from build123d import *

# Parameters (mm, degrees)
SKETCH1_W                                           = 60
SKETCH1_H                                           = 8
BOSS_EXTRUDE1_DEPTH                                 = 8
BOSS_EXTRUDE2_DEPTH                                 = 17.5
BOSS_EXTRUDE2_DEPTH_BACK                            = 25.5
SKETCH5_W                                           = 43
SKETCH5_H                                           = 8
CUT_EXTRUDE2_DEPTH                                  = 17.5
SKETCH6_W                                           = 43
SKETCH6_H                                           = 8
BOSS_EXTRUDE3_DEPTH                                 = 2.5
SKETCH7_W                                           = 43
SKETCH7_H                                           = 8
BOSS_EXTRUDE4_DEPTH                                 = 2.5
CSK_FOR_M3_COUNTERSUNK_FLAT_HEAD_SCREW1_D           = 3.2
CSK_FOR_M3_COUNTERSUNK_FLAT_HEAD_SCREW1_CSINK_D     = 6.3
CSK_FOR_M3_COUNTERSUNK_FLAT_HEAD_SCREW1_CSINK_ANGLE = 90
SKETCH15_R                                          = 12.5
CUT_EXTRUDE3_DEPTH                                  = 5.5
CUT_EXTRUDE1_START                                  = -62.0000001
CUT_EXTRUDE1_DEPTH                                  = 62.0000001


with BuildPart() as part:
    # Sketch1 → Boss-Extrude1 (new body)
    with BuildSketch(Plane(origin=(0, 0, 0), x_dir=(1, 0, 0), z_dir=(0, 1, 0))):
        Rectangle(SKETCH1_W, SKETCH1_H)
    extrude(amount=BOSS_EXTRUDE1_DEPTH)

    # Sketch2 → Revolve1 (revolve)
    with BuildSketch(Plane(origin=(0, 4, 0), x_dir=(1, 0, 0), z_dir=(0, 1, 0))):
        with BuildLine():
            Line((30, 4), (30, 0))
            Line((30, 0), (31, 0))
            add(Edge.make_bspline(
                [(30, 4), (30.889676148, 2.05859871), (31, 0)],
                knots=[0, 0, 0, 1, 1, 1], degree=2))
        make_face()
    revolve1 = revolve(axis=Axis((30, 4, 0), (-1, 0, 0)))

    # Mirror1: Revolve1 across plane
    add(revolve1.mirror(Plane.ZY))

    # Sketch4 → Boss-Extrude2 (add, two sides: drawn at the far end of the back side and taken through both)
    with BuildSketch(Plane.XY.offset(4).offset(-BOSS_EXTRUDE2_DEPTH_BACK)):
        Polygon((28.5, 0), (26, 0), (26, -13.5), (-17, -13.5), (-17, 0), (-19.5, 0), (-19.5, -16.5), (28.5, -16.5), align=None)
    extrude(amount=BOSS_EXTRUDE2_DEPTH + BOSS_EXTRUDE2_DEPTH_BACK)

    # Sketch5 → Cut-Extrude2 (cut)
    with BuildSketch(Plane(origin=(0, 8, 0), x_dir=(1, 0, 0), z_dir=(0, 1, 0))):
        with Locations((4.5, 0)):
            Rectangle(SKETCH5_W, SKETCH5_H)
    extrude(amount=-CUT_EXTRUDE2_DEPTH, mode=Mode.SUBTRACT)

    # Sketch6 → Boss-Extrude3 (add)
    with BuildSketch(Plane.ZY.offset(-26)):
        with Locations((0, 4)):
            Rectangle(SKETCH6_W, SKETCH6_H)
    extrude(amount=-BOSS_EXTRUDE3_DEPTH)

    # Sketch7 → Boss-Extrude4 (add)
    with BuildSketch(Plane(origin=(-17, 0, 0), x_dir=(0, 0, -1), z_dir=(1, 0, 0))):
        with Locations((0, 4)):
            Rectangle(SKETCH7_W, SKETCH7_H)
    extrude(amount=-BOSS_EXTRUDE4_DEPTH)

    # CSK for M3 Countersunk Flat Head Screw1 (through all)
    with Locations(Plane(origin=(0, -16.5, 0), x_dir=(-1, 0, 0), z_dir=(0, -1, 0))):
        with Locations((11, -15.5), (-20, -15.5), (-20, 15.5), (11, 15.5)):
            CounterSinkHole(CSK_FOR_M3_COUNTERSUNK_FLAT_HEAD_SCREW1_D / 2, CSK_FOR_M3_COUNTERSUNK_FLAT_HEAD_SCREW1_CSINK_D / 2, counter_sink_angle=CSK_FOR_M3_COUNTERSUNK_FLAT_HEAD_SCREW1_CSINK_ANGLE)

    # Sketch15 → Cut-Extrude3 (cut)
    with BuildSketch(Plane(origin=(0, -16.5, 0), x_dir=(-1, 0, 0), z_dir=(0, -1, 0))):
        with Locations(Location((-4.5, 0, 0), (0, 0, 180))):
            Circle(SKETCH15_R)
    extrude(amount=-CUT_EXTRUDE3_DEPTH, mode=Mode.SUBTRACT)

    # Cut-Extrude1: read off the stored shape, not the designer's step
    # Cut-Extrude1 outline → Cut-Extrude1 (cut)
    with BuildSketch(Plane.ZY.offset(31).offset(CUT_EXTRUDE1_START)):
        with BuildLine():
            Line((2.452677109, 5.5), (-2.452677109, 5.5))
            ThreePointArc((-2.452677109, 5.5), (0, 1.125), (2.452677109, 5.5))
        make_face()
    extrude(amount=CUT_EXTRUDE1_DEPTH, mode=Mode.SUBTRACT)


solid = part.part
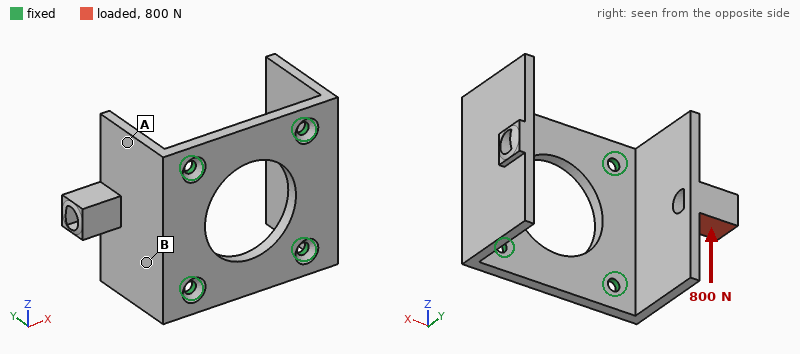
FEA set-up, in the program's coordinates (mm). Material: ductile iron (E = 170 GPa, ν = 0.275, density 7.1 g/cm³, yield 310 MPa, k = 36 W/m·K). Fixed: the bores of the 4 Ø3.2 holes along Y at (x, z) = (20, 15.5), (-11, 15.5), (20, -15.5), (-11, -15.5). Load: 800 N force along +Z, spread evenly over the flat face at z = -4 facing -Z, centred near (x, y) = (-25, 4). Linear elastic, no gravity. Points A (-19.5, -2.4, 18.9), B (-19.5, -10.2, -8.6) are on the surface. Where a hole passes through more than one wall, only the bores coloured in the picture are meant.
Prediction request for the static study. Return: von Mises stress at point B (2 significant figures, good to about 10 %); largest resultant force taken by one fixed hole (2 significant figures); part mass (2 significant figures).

56 MPa
670 N
68 g
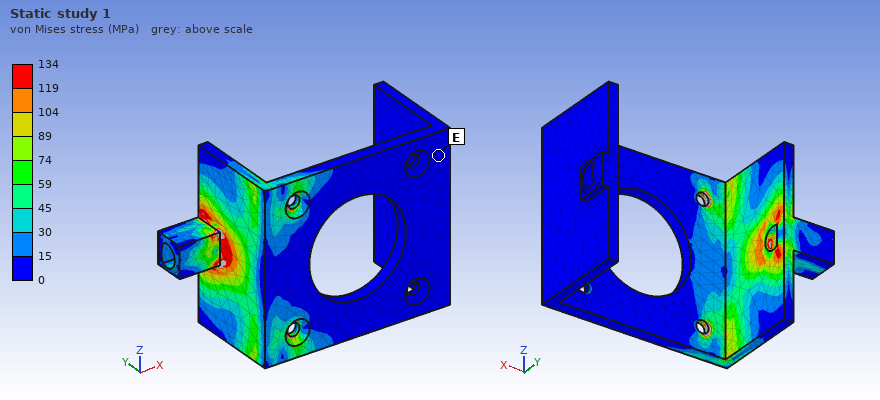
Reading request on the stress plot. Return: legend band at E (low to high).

0 to 15 MPa
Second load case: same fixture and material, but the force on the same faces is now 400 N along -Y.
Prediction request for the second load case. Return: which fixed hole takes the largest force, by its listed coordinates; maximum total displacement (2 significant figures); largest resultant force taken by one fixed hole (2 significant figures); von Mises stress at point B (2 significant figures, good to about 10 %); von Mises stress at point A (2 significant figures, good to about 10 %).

(-11, -15.5)
0.19 mm
320 N
58 MPa
44 MPa
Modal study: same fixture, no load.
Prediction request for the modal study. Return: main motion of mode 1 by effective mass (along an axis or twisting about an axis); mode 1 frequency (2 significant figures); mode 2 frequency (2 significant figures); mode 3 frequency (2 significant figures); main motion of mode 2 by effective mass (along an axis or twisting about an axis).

along X
2100 Hz
2500 Hz
5000 Hz
along X
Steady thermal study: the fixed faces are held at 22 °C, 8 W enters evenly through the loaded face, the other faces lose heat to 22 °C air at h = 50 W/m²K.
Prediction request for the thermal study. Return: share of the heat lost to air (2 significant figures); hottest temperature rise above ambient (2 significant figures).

54 %
81 K
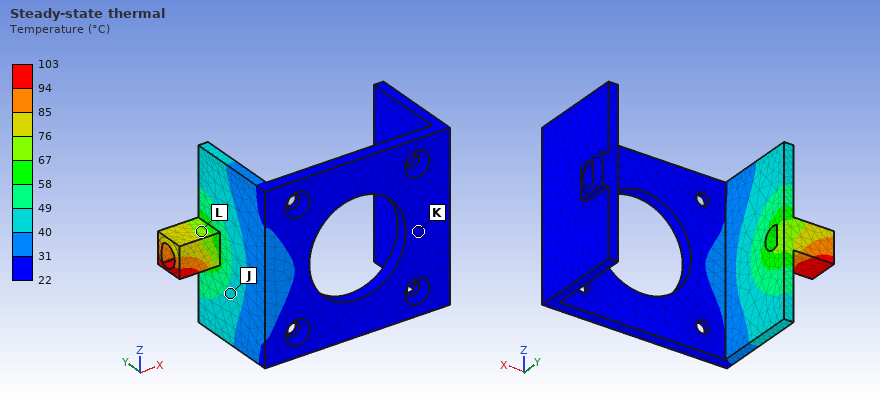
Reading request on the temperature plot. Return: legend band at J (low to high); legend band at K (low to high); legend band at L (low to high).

40 to 49 °C
22 to 31 °C
67 to 76 °C
